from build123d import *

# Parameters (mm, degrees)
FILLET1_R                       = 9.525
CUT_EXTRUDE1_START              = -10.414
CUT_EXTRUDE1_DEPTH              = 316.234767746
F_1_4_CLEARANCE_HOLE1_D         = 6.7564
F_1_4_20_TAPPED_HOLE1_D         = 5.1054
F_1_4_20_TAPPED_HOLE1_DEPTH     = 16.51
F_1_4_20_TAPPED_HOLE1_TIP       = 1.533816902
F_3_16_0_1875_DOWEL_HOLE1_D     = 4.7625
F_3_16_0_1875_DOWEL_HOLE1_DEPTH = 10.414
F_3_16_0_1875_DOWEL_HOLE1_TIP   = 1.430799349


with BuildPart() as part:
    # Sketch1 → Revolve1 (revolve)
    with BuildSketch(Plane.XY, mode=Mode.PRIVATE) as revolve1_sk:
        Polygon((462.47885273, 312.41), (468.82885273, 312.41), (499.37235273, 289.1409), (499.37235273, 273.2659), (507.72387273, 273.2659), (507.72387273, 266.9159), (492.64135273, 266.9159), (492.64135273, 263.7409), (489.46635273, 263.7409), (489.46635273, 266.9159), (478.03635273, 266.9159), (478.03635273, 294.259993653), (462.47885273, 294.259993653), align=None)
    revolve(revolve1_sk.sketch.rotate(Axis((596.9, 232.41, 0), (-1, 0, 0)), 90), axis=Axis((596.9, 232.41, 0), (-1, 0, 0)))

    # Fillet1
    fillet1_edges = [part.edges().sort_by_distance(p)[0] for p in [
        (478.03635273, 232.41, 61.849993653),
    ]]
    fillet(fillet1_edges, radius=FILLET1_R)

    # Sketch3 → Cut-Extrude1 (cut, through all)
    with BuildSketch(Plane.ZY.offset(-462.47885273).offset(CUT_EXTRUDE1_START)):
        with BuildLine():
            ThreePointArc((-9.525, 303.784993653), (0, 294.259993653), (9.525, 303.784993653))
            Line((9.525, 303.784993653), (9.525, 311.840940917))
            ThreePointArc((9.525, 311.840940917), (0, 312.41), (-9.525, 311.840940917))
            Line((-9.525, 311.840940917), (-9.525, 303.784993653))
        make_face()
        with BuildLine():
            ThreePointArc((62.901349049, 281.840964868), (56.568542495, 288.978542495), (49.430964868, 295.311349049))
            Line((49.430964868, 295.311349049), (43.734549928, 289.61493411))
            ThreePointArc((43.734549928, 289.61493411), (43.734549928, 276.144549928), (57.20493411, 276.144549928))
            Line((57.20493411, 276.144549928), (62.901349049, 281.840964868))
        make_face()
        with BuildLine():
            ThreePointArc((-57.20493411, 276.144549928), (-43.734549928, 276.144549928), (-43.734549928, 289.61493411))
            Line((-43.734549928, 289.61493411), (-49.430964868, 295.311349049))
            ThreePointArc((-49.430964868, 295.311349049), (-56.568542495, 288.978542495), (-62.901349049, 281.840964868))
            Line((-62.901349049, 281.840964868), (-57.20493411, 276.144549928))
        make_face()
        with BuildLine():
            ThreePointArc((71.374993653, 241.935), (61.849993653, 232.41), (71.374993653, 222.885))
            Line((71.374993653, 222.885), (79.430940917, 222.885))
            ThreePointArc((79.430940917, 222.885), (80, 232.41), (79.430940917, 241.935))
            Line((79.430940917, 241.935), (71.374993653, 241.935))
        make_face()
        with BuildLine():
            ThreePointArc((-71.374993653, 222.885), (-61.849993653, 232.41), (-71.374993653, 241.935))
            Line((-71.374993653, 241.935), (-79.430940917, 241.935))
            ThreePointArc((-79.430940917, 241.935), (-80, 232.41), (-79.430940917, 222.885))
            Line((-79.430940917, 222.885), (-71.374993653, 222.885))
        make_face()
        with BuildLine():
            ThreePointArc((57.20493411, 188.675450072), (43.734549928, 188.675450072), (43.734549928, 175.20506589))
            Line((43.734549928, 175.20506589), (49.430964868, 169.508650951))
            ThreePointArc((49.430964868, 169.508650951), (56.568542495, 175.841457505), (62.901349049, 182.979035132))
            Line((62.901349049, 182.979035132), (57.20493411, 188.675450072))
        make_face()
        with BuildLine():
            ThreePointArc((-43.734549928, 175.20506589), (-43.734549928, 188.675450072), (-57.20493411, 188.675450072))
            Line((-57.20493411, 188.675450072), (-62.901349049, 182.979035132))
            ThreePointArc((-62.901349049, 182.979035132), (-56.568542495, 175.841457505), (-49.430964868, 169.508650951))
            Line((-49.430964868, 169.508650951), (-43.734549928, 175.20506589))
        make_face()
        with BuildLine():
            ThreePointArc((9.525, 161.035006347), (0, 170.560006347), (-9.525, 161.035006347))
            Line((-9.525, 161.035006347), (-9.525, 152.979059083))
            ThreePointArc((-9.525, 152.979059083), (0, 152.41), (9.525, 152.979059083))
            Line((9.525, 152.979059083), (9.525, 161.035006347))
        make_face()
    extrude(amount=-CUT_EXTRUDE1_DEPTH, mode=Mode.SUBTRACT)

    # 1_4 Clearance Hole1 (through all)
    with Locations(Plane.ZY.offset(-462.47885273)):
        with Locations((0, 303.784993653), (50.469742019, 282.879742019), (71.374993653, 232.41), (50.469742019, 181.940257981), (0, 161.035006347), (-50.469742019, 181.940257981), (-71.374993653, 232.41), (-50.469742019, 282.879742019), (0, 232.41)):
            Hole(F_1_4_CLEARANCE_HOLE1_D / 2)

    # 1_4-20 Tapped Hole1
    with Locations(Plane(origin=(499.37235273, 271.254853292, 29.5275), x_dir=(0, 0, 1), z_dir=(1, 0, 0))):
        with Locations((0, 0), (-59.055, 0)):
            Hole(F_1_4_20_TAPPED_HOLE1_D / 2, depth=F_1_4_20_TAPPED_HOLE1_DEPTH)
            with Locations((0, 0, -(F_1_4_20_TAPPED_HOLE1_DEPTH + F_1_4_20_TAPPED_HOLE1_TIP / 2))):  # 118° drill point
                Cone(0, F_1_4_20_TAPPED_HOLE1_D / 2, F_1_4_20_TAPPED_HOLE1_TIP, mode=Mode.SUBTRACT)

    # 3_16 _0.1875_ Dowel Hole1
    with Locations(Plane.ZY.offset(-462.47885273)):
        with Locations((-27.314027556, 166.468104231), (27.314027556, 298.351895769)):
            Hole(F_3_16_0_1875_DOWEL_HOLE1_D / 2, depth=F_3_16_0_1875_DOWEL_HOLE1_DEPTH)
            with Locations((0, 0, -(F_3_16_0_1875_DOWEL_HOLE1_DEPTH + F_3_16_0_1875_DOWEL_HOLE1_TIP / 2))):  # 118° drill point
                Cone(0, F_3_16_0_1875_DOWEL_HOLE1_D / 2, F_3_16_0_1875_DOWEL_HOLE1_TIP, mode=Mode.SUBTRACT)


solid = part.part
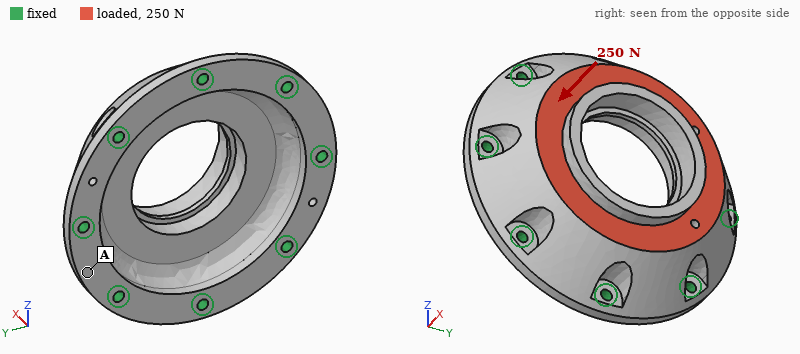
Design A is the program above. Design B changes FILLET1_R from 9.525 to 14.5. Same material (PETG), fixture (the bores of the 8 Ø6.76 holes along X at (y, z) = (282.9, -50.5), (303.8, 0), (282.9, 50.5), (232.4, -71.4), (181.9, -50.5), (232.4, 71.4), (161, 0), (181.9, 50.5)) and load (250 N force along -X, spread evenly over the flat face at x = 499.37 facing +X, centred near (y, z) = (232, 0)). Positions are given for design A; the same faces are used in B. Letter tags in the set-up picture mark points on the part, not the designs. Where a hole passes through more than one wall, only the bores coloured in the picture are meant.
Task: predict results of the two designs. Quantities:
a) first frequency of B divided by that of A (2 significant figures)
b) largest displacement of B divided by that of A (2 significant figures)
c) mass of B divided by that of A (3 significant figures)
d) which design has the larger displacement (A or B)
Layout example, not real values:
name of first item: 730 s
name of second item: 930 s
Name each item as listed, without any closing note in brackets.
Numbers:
first frequency of B divided by that of A: 1.0
largest displacement of B divided by that of A: 0.87
mass of B divided by that of A: 1.03
which design has the larger displacement: A
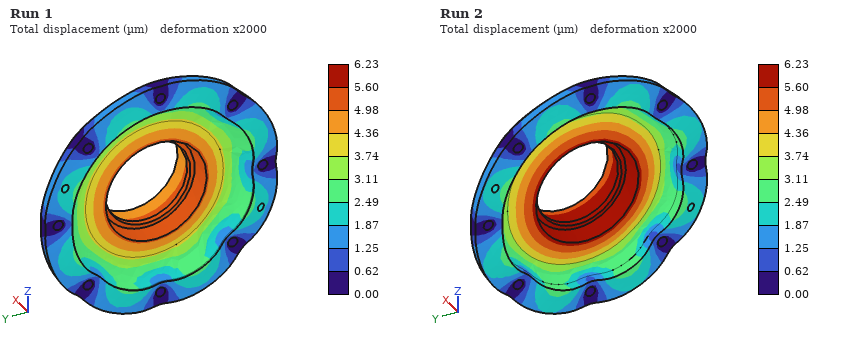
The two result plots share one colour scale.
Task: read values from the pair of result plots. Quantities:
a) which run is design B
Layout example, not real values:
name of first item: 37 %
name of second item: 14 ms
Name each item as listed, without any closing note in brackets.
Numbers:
which run is design B: Run 1
